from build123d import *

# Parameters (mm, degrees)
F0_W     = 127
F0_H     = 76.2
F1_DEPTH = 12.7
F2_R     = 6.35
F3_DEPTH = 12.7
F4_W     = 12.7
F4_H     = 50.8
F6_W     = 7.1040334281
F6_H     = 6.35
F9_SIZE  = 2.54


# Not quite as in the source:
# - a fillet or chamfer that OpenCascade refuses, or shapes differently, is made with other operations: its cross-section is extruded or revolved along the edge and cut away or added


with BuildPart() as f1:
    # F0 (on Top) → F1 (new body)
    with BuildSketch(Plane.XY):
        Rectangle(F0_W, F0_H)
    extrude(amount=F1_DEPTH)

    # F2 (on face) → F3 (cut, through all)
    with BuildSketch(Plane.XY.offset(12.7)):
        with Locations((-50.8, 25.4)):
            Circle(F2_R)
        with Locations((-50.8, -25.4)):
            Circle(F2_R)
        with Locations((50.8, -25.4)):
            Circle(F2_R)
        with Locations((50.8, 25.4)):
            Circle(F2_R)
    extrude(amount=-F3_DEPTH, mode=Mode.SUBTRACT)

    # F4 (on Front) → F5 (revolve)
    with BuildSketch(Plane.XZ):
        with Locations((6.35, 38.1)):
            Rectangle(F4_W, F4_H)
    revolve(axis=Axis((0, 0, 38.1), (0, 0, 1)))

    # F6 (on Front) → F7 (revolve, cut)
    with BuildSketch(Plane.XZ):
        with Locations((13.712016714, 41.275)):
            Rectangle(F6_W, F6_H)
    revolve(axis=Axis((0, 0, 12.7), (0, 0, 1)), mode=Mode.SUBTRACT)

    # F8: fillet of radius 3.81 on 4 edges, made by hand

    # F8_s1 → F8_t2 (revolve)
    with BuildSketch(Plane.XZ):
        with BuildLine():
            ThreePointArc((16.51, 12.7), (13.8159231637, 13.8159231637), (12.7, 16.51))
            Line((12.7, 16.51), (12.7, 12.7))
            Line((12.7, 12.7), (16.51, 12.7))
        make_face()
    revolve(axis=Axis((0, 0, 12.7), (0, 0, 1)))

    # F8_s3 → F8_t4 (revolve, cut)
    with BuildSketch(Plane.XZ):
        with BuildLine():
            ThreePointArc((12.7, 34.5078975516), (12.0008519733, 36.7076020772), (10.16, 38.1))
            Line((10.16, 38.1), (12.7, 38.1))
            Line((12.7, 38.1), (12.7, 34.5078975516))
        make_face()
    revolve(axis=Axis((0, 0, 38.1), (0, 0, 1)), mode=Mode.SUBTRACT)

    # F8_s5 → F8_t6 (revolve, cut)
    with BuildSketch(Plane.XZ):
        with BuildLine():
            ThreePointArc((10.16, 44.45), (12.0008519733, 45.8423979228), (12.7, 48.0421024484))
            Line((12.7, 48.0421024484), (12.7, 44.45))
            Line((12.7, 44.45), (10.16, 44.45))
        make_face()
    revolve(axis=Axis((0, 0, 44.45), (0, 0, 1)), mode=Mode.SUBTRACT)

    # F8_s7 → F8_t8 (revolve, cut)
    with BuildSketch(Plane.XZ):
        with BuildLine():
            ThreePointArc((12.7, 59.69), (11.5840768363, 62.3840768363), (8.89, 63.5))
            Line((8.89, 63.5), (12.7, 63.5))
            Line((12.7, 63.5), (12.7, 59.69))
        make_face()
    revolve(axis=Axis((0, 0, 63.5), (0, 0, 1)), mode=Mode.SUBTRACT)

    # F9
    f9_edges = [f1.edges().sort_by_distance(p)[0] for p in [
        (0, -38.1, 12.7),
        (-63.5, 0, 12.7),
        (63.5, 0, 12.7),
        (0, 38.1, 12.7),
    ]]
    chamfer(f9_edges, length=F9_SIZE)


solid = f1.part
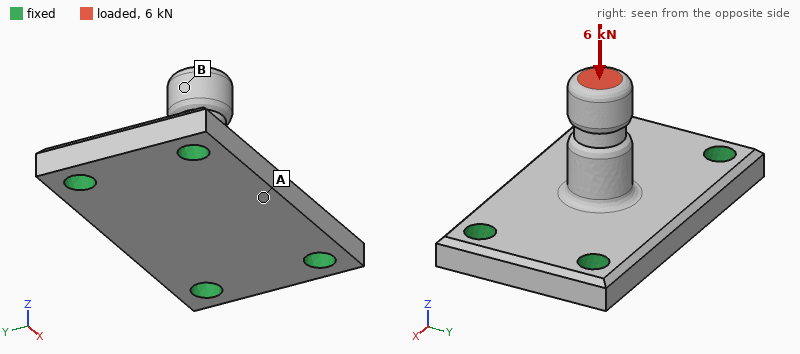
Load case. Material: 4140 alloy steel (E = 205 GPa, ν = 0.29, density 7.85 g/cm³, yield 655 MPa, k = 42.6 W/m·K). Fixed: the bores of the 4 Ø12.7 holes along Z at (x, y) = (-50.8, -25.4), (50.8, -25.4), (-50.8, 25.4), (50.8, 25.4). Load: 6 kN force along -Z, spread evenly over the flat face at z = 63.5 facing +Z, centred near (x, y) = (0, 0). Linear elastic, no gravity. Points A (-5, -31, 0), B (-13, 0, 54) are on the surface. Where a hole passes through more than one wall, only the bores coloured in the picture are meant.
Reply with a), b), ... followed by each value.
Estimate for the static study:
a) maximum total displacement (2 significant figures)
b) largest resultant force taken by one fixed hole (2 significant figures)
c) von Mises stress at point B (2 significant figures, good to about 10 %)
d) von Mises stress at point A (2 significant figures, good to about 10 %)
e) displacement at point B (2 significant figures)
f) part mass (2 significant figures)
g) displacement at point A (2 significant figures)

a) 15 µm
b) 1.5 kN
c) 8.5 MPa
d) 19 MPa
e) 14 µm
f) 1.1 kg
g) 8.8 µm
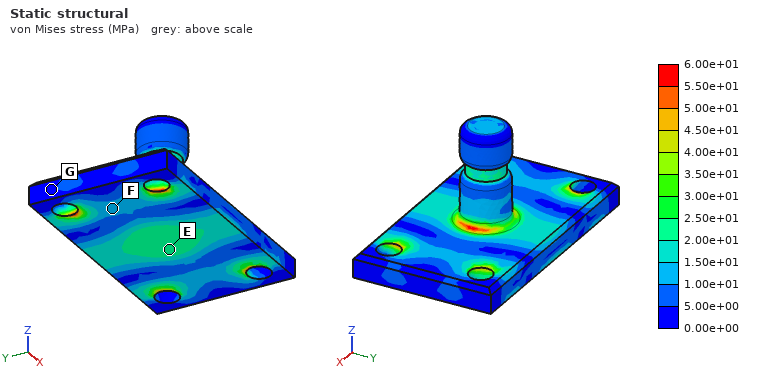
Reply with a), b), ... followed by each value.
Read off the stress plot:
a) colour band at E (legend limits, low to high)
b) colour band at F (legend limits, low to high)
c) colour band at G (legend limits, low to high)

a) 2.00e+01 to 2.50e+01 MPa
b) 1.00e+01 to 1.50e+01 MPa
c) 0.00e+00 to 5.00e+00 MPa
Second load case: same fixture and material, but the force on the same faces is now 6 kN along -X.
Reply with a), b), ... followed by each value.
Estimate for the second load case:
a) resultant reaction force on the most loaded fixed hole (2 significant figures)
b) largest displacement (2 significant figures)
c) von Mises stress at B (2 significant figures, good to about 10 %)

a) 2.9 kN
b) 0.13 mm
c) 36 MPa
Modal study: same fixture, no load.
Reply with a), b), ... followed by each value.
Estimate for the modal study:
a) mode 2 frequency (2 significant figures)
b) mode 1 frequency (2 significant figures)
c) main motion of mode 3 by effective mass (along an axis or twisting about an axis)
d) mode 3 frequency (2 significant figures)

a) 4600 Hz
b) 3900 Hz
c) along Z
d) 5200 Hz
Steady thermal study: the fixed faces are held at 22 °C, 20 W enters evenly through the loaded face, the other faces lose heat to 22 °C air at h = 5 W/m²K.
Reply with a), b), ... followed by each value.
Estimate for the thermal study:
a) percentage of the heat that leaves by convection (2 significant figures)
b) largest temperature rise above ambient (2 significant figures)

a) 6.4 %
b) 70 K
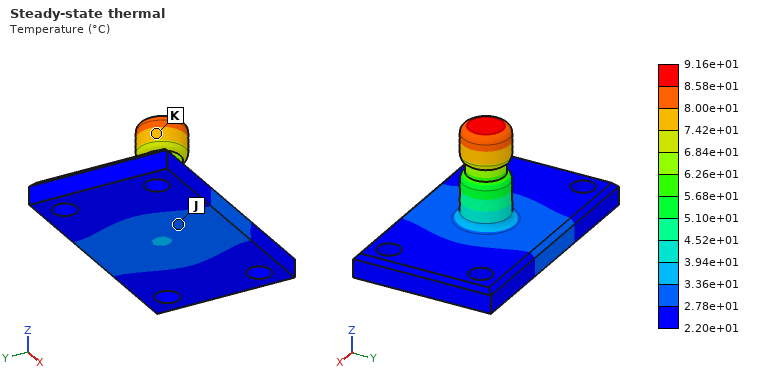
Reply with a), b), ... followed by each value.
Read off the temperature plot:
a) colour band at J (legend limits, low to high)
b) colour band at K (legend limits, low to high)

a) 2.78e+01 to 3.36e+01 °C
b) 7.42e+01 to 8.00e+01 °C
